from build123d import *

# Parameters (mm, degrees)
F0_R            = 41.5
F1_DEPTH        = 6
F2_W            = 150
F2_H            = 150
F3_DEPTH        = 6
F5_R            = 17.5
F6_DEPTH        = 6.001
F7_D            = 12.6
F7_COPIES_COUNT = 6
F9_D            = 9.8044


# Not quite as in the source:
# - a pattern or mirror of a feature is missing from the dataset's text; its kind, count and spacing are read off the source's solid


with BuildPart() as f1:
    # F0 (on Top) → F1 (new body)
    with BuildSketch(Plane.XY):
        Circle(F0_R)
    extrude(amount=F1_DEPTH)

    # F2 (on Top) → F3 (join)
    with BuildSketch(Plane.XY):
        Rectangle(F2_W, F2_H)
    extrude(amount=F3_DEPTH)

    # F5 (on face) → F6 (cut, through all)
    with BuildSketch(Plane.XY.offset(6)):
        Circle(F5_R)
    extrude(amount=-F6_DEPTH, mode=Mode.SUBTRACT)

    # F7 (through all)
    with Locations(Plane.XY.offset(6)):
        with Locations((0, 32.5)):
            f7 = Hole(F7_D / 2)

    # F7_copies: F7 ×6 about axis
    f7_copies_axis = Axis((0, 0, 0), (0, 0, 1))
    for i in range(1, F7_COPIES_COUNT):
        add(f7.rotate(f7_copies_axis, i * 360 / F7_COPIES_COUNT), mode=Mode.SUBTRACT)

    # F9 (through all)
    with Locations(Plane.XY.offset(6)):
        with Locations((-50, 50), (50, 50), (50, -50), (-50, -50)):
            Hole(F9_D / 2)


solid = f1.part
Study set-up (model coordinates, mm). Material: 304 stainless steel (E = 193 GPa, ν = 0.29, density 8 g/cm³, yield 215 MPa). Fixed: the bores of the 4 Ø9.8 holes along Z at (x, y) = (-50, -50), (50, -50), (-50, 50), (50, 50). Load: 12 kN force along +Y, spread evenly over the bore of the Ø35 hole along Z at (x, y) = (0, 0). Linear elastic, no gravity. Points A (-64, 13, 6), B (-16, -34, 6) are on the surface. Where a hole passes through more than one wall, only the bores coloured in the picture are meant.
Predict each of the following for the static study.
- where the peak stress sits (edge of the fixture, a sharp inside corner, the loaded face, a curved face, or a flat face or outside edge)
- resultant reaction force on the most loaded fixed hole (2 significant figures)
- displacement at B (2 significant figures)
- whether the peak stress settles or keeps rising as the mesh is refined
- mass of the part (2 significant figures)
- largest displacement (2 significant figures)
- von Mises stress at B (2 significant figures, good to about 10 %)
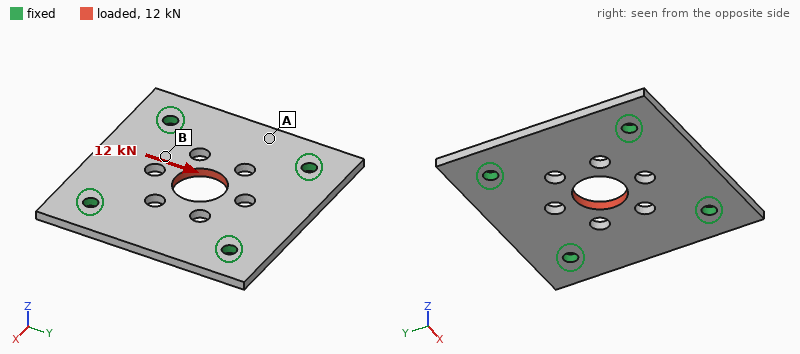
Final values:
edge of the fixture
3.2 kN
4.7 µm
keeps rising
980 g
7.5 µm
16 MPa
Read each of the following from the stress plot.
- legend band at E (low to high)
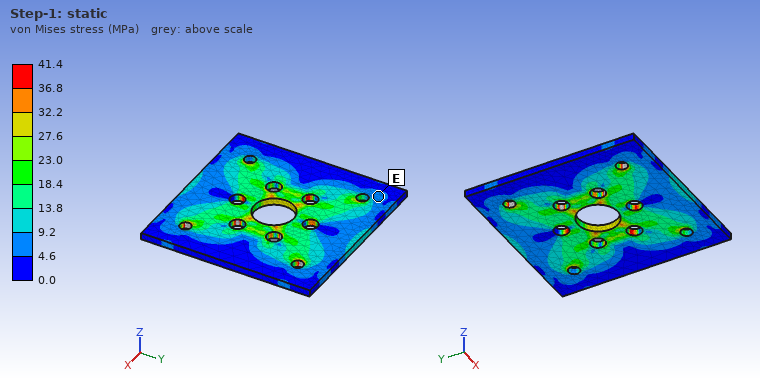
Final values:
4.6 to 9.2 MPa
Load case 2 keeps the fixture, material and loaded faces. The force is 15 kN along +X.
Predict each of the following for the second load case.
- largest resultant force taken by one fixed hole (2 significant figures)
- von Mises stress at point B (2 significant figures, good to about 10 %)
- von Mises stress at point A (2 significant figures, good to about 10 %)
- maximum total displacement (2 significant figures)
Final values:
4.0 kN
18 MPa
10 MPa
9.4 µm
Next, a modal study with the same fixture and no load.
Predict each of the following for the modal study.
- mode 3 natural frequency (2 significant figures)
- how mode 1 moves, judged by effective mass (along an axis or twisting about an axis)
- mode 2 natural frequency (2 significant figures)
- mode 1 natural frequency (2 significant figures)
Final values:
3100 Hz
along Z
3000 Hz
2400 Hz
